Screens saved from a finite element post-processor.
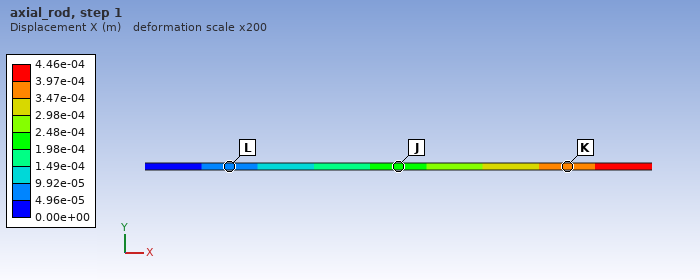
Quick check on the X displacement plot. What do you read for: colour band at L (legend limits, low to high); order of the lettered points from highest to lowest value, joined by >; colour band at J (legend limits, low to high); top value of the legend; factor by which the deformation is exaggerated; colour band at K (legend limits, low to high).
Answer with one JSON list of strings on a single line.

["4.96e-05 to 9.92e-05 m", "K > J > L", "1.98e-04 to 2.48e-04 m", "4.46e-04 m", "200", "3.47e-04 to 3.97e-04 m"]
